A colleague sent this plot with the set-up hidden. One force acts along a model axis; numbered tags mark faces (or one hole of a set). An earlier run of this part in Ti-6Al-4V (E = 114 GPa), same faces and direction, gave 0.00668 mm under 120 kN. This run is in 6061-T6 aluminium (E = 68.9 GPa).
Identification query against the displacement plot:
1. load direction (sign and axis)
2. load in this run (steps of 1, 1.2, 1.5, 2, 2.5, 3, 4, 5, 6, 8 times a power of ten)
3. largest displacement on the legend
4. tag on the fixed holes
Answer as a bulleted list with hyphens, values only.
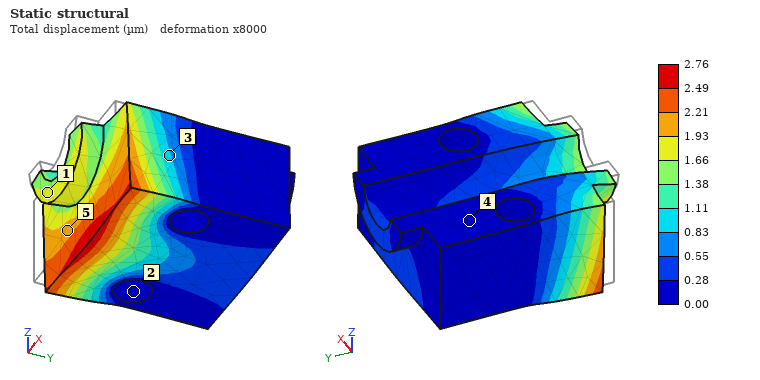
- +Y
- 30 kN
- 2.76 µm
- 2
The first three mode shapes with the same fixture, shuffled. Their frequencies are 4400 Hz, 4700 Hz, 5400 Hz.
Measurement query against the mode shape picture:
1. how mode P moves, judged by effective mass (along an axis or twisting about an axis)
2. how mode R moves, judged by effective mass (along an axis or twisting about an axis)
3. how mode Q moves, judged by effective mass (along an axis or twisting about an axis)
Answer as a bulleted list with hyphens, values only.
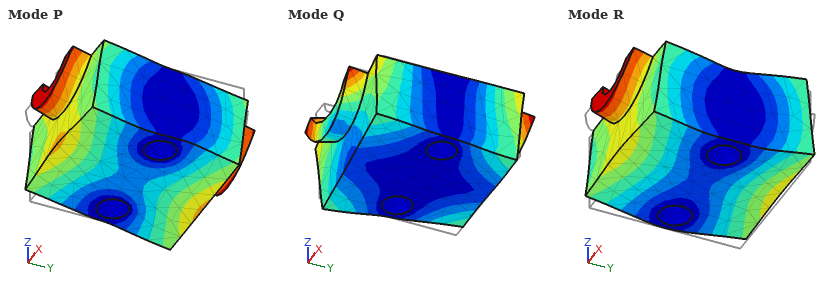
- twisting about X
- along Z
- twisting about Z
